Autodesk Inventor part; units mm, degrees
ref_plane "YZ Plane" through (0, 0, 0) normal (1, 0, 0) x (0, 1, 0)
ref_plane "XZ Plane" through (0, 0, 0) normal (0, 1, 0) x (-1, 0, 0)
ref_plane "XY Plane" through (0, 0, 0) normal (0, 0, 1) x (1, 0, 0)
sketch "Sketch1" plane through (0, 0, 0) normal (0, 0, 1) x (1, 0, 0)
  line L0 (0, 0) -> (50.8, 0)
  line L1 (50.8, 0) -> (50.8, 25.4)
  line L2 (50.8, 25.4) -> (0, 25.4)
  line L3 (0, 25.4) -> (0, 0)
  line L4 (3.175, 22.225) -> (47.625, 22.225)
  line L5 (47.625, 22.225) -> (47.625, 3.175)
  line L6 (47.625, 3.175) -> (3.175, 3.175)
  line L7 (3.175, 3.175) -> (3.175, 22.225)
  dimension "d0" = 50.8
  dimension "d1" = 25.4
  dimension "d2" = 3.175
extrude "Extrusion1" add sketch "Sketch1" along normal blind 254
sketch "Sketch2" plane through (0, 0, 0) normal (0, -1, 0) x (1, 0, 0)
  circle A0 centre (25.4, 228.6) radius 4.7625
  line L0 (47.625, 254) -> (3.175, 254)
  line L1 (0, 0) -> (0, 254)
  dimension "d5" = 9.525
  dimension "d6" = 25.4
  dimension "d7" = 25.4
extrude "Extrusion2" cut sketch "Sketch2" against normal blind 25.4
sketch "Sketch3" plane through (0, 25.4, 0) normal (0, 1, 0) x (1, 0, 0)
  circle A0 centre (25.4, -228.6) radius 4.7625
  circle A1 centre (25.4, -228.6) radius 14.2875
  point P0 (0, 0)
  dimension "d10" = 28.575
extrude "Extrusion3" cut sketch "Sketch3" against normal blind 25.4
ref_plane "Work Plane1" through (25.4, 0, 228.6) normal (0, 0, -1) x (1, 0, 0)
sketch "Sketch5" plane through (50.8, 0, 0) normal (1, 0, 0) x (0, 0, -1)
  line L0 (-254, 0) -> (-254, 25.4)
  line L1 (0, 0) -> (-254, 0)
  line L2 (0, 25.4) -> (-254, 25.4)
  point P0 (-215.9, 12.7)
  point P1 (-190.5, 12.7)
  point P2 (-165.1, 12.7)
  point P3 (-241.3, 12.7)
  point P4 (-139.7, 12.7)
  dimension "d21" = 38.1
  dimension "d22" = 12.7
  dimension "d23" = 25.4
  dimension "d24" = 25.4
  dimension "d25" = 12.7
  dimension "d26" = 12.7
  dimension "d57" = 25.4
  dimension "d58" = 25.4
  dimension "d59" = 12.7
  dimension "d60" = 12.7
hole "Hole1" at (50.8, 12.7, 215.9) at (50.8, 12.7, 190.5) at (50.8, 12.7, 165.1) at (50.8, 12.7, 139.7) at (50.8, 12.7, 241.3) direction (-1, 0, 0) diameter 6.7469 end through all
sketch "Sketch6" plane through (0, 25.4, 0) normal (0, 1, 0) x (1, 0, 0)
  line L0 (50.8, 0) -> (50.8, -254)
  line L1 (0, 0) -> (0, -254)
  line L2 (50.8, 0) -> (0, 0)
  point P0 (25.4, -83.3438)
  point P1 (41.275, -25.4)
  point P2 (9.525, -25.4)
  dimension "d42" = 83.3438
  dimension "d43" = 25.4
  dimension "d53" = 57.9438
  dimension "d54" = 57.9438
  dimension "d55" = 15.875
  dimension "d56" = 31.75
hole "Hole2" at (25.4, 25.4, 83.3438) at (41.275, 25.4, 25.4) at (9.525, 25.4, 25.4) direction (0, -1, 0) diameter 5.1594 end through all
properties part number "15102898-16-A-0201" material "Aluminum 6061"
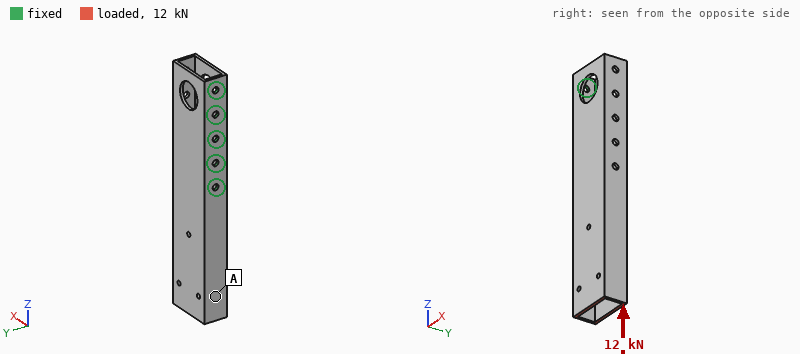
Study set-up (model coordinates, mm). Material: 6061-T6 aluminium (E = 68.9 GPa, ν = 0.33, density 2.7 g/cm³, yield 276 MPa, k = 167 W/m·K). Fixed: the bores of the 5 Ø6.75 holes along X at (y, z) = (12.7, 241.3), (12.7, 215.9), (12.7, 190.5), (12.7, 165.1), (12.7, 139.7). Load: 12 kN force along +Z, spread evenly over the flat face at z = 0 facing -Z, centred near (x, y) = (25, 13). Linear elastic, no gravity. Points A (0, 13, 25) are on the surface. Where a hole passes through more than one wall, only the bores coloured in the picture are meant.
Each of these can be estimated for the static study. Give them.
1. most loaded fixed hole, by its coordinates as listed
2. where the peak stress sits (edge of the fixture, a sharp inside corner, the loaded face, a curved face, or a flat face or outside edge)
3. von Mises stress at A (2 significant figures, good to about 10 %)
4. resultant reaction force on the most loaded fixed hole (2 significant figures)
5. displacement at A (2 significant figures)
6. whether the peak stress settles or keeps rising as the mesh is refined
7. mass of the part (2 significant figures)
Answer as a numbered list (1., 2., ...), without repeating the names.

1. (12.7, 139.7)
2. edge of the fixture
3. 27 MPa
4. 5.2 kN
5. 0.26 mm
6. keeps rising
7. 290 g
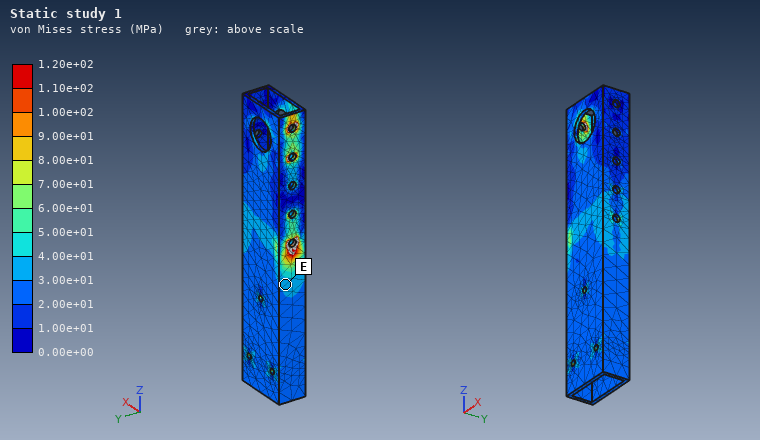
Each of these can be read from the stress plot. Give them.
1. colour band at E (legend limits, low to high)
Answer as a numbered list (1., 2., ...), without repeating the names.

1. 3.00e+01 to 4.00e+01 MPa
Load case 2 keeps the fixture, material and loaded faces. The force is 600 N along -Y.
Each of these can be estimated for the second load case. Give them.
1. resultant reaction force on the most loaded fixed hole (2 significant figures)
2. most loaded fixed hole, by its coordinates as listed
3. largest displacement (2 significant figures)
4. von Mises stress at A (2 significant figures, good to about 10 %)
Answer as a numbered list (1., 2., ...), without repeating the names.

1. 1.8 kN
2. (12.7, 139.7)
3. 0.53 mm
4. 7.4 MPa
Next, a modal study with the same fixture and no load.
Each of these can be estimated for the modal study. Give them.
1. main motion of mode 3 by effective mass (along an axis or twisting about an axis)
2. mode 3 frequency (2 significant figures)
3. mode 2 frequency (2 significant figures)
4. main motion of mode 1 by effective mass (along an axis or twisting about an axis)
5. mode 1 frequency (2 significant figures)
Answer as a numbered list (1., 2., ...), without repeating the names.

1. along X
2. 1100 Hz
3. 1000 Hz
4. along Y
5. 660 Hz
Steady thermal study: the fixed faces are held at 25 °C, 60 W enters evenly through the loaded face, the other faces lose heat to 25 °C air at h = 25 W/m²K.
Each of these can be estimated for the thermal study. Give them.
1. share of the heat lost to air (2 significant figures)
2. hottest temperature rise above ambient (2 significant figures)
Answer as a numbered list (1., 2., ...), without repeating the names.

1. 64 %
2. 77 K
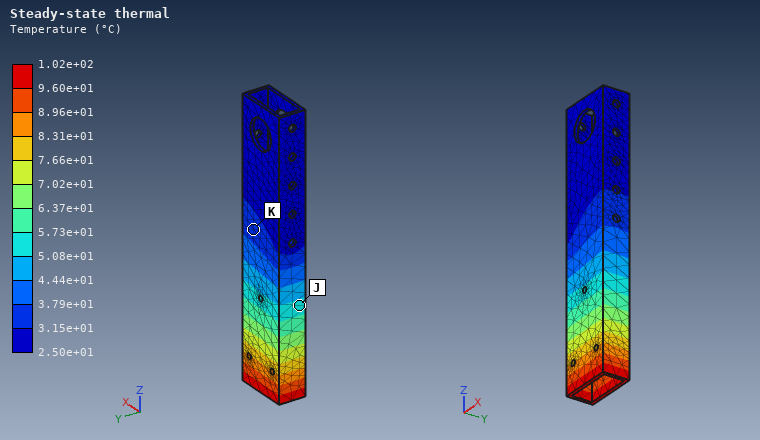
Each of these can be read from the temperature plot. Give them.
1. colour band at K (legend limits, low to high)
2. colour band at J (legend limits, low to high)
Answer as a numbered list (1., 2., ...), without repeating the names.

1. 3.15e+01 to 3.79e+01 °C
2. 5.08e+01 to 5.73e+01 °C
